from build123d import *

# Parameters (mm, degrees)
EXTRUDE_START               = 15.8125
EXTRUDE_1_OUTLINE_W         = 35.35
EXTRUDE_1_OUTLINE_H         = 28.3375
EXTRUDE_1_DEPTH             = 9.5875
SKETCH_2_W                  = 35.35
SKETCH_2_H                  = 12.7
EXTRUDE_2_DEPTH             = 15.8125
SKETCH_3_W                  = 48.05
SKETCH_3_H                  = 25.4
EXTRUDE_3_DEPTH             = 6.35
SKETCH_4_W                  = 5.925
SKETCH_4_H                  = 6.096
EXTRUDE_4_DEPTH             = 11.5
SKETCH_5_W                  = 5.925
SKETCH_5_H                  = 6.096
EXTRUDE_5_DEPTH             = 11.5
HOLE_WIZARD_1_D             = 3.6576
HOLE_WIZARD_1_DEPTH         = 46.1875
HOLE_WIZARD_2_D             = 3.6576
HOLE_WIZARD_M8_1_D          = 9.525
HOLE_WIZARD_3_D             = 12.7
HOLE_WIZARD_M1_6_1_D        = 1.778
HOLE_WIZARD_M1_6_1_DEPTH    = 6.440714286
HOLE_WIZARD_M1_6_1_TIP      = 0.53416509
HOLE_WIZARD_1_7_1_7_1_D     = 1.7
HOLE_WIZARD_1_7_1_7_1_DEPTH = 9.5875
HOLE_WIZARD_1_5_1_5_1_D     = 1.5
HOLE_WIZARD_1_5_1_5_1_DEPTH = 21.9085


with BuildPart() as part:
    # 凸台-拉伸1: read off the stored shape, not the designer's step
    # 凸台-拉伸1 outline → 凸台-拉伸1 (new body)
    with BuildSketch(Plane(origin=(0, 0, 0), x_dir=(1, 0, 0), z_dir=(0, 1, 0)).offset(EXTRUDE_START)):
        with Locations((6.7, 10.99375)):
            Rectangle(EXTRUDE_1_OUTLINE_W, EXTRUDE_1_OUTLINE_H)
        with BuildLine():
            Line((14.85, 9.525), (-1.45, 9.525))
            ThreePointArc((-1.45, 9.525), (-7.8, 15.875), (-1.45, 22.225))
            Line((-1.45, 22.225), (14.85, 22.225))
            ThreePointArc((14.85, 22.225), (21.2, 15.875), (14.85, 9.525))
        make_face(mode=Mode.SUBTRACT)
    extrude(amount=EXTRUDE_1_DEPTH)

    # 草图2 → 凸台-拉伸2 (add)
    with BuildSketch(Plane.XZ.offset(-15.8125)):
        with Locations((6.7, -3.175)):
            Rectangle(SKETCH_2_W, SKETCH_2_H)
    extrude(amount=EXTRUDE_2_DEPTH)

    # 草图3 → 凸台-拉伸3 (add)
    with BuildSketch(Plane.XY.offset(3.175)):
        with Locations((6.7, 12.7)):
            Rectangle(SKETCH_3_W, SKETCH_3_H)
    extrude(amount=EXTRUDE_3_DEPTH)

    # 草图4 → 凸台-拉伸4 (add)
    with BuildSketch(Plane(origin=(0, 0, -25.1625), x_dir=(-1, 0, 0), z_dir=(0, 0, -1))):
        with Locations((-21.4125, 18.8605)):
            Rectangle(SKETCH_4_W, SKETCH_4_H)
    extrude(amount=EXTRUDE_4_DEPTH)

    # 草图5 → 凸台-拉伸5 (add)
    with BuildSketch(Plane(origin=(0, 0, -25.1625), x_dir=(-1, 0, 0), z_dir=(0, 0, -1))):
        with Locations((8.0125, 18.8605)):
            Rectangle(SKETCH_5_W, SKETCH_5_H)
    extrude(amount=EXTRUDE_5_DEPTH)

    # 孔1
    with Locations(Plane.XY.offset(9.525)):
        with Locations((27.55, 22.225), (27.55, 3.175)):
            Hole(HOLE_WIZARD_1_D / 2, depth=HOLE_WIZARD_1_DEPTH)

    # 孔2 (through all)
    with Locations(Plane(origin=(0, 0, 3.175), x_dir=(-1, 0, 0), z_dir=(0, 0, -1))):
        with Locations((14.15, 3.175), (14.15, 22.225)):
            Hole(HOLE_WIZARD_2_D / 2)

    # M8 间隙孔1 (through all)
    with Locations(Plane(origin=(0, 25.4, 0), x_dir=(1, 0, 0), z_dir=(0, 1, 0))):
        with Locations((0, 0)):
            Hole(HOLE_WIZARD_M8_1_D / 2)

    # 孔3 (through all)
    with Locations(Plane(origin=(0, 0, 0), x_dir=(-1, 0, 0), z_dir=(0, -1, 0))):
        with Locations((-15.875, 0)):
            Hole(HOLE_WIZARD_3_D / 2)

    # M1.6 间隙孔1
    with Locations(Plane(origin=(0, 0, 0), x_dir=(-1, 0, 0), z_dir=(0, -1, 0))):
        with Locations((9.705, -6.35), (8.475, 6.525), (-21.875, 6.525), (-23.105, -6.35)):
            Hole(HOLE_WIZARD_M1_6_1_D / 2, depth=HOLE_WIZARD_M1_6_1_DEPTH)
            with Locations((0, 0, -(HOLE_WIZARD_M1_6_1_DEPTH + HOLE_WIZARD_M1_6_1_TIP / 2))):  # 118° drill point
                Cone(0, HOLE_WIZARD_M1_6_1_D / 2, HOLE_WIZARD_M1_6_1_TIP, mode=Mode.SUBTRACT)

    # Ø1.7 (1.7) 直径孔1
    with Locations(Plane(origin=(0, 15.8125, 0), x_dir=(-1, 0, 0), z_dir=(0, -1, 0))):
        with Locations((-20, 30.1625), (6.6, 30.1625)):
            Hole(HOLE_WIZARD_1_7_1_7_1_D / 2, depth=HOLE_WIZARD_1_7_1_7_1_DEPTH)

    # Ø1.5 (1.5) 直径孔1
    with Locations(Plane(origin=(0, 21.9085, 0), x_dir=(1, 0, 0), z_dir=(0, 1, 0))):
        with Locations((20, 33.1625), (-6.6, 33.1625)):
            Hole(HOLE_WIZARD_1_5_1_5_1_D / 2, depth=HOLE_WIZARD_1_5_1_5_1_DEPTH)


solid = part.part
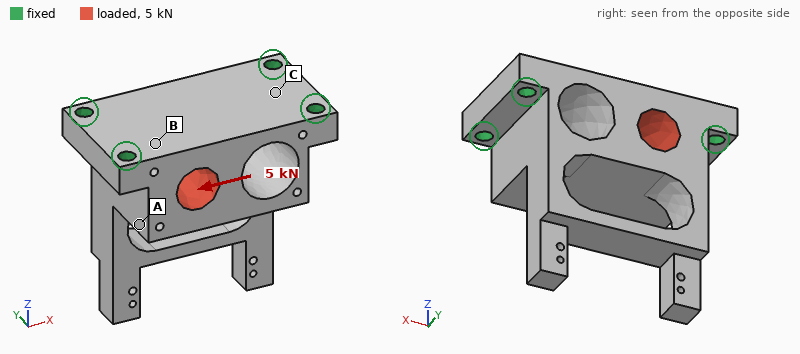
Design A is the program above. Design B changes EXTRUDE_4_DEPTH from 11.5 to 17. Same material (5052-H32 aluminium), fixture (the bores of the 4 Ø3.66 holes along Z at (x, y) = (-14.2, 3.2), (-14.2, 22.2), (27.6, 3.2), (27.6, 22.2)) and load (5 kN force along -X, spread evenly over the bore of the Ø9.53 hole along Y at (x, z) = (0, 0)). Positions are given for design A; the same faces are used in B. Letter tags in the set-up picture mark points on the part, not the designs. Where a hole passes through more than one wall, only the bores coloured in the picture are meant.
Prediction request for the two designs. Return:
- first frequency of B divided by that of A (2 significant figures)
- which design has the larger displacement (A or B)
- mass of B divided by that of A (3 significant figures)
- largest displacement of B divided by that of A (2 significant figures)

0.83
B
1.01
1.1
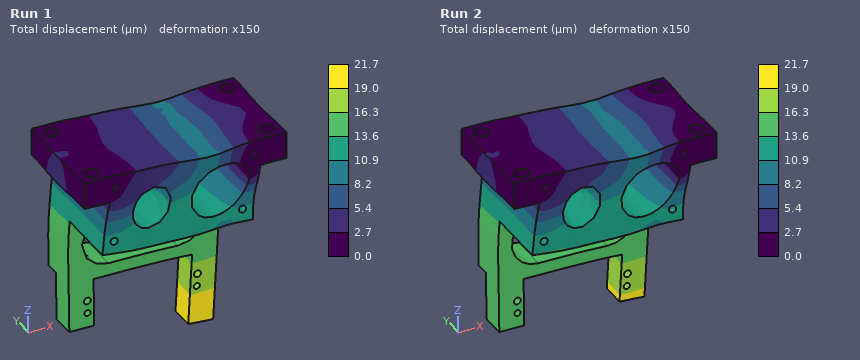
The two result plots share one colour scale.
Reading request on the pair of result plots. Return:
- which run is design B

Run 1
